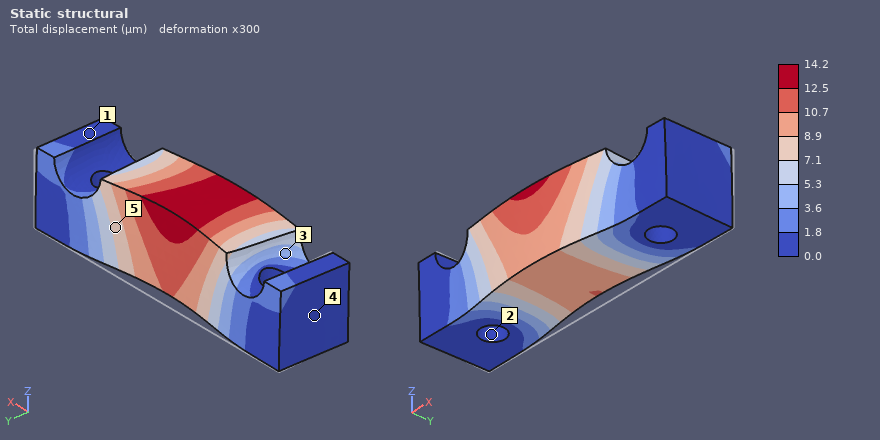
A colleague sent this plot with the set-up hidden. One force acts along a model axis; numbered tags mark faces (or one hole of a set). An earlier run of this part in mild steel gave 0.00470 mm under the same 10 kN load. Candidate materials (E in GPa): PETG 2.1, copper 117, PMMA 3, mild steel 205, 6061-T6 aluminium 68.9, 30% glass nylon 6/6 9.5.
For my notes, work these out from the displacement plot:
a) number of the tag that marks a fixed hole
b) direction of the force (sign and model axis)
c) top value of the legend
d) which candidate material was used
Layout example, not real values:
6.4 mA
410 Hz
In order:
2
-Y
14.2 µm
6061-T6 aluminium
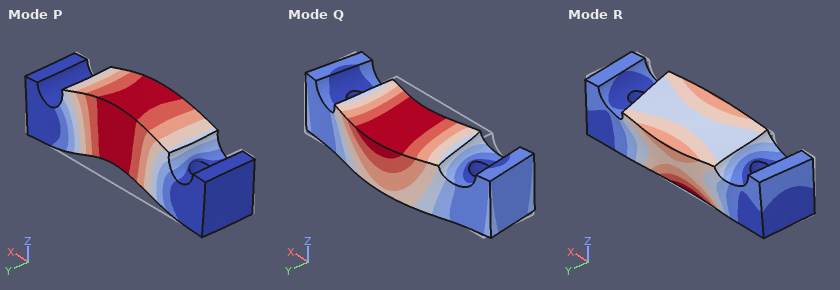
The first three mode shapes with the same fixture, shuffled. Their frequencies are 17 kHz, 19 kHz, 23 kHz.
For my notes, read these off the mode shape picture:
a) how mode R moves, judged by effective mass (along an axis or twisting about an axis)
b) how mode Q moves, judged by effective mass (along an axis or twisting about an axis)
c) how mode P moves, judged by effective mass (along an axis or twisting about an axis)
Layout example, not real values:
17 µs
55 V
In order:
twisting about X
along Y
along Z
